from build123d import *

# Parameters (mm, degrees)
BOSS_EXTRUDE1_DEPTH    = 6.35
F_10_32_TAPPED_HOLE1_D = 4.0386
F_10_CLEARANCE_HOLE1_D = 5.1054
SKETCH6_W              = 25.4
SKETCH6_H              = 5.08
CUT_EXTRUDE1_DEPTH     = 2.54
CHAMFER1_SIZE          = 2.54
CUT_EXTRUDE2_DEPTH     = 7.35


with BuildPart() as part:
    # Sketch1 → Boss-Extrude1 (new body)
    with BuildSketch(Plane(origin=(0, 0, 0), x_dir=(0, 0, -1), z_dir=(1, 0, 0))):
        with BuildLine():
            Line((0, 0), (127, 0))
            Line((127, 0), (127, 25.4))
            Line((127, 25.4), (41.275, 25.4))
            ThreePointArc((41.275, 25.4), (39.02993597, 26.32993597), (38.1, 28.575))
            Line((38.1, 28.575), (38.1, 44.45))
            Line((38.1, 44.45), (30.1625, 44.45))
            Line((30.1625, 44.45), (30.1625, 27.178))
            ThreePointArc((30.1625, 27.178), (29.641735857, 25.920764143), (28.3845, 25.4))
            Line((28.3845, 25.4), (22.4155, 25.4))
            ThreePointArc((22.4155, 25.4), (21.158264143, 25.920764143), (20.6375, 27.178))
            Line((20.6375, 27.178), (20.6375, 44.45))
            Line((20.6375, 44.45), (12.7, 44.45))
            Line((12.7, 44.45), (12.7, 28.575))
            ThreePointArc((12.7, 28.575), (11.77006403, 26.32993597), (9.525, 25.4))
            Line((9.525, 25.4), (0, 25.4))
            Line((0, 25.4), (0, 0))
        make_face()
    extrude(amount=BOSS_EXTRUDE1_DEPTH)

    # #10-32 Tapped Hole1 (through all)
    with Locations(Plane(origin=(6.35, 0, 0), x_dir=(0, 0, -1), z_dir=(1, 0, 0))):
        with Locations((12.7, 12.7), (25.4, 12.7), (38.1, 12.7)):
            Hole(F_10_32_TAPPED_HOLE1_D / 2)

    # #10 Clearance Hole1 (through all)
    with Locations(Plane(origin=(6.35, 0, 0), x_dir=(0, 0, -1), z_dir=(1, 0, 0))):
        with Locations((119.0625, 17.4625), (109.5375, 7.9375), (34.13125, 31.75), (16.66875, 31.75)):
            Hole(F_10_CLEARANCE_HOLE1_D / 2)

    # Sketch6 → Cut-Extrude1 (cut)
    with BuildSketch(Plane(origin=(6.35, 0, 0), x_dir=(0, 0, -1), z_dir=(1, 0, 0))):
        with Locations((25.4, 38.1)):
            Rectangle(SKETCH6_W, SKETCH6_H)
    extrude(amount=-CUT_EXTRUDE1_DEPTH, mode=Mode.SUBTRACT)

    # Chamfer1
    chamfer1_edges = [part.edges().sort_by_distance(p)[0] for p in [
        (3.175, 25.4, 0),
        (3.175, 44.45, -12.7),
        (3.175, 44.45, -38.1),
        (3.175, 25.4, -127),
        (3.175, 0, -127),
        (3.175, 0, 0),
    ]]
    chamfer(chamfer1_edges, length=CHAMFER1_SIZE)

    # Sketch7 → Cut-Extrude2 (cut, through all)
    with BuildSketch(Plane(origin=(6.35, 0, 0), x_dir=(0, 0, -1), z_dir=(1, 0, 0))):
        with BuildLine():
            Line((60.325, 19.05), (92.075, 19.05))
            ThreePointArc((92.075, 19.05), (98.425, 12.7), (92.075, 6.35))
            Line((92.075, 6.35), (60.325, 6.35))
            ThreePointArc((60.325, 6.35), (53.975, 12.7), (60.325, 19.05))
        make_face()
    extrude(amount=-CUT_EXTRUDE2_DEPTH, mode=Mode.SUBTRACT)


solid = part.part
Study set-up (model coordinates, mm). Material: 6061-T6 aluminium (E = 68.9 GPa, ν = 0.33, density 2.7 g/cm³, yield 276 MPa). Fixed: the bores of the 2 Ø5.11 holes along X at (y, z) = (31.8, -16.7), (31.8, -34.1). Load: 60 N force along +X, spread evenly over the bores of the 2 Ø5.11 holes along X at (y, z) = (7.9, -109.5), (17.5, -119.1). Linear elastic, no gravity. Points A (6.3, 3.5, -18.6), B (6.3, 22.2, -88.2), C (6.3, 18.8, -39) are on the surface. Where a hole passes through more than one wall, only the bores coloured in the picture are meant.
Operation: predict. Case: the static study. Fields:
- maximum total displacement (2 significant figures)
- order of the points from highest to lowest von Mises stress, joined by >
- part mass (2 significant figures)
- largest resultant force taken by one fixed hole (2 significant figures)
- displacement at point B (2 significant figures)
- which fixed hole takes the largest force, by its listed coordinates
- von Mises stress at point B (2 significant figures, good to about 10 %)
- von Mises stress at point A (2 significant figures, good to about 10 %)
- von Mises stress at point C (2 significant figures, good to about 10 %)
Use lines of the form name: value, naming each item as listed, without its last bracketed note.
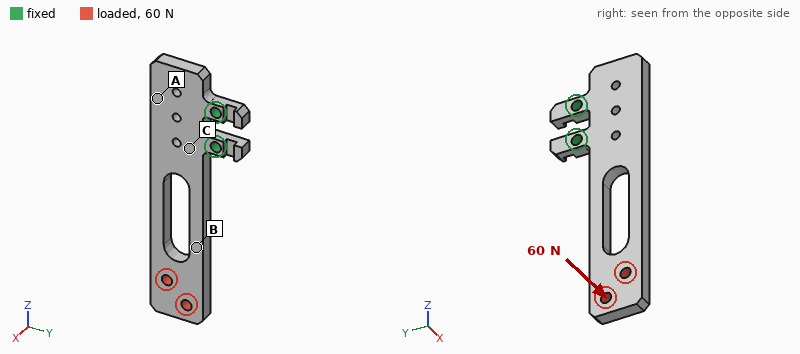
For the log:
maximum total displacement: 0.63 mm
order of the points from highest to lowest von Mises stress, joined by >: C > B > A
part mass: 49 g
largest resultant force taken by one fixed hole: 220 N
displacement at point B: 0.27 mm
which fixed hole takes the largest force, by its listed coordinates: (31.8, -34.1)
von Mises stress at point B: 18 MPa
von Mises stress at point A: 8.1 MPa
von Mises stress at point C: 30 MPa
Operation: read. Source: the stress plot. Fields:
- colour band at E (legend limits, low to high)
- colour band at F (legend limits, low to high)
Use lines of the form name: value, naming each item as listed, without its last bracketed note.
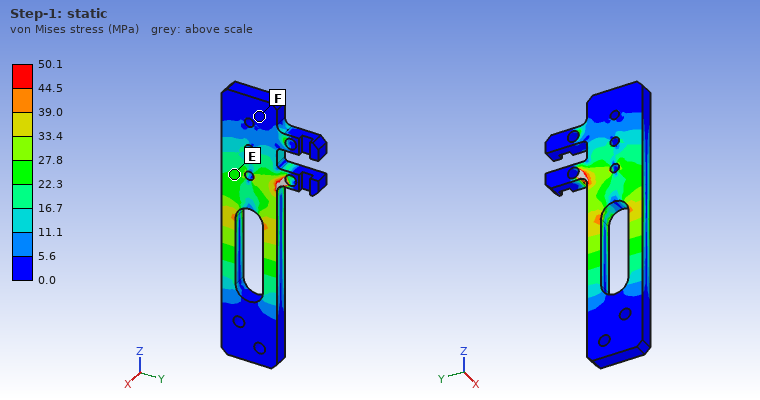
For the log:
colour band at E: 22.3 to 27.8 MPa
colour band at F: 0.0 to 5.6 MPa
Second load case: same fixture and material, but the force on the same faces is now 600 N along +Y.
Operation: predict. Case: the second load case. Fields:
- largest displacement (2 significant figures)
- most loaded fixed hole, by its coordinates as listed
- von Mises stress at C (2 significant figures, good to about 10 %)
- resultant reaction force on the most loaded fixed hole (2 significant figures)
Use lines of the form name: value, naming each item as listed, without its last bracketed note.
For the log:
largest displacement: 0.62 mm
most loaded fixed hole, by its coordinates as listed: (31.8, -34.1)
von Mises stress at C: 22 MPa
resultant reaction force on the most loaded fixed hole: 3.0 kN
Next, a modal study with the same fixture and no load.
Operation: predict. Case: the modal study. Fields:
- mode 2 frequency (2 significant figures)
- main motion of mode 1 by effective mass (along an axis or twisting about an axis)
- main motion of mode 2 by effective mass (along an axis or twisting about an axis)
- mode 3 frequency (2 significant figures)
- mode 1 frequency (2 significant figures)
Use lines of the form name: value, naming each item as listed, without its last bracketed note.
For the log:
mode 2 frequency: 1400 Hz
main motion of mode 1 by effective mass: along X
main motion of mode 2 by effective mass: along Y
mode 3 frequency: 2300 Hz
mode 1 frequency: 480 Hz
